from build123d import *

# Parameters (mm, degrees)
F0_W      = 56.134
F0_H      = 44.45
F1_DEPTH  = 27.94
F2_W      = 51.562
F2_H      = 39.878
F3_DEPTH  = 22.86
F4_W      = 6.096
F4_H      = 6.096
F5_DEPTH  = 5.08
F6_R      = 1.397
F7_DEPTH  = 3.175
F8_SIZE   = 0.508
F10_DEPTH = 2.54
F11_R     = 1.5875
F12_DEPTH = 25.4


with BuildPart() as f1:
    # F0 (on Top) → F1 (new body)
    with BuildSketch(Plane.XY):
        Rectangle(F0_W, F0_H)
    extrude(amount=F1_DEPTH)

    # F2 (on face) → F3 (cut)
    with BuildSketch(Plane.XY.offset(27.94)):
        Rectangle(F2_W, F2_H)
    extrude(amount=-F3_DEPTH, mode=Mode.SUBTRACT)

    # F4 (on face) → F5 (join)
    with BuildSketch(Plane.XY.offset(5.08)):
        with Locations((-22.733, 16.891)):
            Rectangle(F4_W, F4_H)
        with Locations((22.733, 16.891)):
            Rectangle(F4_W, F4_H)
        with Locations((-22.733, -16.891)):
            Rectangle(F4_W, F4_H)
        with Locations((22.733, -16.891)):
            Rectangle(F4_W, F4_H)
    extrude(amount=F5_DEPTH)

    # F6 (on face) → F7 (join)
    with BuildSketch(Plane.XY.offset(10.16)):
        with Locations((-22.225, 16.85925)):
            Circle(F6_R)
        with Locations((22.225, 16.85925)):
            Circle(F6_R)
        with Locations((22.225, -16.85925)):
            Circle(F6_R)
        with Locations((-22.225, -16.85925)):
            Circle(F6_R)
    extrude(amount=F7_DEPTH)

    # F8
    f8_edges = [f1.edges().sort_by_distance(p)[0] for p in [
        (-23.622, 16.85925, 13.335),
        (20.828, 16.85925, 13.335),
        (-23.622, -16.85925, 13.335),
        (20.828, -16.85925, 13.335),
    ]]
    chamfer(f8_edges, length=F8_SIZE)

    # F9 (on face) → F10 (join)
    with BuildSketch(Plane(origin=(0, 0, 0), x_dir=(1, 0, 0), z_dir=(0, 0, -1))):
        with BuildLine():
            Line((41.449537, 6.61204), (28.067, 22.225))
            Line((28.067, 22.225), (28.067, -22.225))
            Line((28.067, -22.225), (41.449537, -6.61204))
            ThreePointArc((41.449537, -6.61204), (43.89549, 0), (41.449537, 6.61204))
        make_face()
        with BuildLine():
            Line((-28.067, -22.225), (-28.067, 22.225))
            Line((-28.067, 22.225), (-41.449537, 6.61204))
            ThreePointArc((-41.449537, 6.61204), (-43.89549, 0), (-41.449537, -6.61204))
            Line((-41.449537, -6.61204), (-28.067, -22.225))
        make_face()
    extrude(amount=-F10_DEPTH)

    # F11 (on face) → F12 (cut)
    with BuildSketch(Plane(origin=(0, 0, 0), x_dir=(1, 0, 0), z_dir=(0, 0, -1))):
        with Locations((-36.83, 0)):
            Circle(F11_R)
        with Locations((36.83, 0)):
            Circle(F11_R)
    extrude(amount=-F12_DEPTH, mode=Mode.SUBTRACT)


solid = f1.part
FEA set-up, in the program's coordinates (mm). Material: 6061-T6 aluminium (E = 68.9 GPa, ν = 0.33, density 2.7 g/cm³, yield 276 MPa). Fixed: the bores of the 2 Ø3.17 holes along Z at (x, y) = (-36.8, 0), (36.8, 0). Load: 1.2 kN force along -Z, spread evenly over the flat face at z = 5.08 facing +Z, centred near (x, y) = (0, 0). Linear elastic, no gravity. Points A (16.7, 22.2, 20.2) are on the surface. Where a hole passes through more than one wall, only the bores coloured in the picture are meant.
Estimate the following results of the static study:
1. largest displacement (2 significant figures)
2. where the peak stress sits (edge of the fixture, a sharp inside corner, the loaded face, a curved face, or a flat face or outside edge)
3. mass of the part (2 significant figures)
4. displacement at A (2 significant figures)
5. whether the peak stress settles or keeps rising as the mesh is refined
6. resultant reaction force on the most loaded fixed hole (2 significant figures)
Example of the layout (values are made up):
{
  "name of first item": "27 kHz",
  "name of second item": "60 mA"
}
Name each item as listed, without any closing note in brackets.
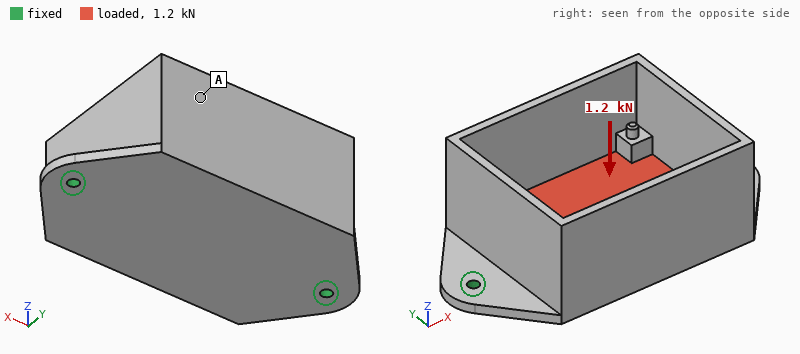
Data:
{
  "largest displacement": "61 µm",
  "where the peak stress sits": "edge of the fixture",
  "mass of the part": "69 g",
  "displacement at A": "47 µm",
  "whether the peak stress settles or keeps rising as the mesh is refined": "keeps rising",
  "resultant reaction force on the most loaded fixed hole": "730 N"
}
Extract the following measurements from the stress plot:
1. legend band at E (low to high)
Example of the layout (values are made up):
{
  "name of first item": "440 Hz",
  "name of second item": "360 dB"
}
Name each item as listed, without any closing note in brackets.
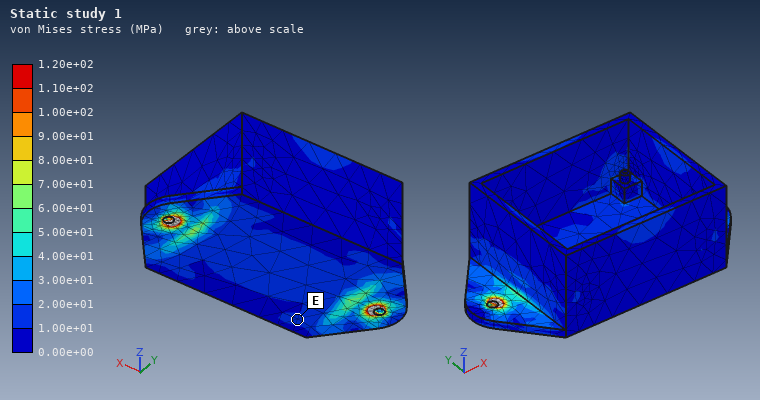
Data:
{
  "legend band at E": "1.00e+01 to 2.00e+01 MPa"
}
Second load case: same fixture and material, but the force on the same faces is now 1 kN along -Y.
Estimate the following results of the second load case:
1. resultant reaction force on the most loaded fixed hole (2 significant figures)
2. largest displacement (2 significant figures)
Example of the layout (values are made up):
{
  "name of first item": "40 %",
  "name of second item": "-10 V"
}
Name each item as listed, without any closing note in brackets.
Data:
{
  "resultant reaction force on the most loaded fixed hole": "500 N",
  "largest displacement": "0.15 mm"
}
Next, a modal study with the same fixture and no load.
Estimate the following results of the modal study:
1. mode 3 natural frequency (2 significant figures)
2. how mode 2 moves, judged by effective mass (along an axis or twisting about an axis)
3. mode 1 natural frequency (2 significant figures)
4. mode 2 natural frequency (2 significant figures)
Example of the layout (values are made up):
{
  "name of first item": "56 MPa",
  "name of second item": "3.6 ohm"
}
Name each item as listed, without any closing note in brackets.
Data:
{
  "mode 3 natural frequency": "3500 Hz",
  "how mode 2 moves, judged by effective mass": "along Z",
  "mode 1 natural frequency": "1000 Hz",
  "mode 2 natural frequency": "3200 Hz"
}
